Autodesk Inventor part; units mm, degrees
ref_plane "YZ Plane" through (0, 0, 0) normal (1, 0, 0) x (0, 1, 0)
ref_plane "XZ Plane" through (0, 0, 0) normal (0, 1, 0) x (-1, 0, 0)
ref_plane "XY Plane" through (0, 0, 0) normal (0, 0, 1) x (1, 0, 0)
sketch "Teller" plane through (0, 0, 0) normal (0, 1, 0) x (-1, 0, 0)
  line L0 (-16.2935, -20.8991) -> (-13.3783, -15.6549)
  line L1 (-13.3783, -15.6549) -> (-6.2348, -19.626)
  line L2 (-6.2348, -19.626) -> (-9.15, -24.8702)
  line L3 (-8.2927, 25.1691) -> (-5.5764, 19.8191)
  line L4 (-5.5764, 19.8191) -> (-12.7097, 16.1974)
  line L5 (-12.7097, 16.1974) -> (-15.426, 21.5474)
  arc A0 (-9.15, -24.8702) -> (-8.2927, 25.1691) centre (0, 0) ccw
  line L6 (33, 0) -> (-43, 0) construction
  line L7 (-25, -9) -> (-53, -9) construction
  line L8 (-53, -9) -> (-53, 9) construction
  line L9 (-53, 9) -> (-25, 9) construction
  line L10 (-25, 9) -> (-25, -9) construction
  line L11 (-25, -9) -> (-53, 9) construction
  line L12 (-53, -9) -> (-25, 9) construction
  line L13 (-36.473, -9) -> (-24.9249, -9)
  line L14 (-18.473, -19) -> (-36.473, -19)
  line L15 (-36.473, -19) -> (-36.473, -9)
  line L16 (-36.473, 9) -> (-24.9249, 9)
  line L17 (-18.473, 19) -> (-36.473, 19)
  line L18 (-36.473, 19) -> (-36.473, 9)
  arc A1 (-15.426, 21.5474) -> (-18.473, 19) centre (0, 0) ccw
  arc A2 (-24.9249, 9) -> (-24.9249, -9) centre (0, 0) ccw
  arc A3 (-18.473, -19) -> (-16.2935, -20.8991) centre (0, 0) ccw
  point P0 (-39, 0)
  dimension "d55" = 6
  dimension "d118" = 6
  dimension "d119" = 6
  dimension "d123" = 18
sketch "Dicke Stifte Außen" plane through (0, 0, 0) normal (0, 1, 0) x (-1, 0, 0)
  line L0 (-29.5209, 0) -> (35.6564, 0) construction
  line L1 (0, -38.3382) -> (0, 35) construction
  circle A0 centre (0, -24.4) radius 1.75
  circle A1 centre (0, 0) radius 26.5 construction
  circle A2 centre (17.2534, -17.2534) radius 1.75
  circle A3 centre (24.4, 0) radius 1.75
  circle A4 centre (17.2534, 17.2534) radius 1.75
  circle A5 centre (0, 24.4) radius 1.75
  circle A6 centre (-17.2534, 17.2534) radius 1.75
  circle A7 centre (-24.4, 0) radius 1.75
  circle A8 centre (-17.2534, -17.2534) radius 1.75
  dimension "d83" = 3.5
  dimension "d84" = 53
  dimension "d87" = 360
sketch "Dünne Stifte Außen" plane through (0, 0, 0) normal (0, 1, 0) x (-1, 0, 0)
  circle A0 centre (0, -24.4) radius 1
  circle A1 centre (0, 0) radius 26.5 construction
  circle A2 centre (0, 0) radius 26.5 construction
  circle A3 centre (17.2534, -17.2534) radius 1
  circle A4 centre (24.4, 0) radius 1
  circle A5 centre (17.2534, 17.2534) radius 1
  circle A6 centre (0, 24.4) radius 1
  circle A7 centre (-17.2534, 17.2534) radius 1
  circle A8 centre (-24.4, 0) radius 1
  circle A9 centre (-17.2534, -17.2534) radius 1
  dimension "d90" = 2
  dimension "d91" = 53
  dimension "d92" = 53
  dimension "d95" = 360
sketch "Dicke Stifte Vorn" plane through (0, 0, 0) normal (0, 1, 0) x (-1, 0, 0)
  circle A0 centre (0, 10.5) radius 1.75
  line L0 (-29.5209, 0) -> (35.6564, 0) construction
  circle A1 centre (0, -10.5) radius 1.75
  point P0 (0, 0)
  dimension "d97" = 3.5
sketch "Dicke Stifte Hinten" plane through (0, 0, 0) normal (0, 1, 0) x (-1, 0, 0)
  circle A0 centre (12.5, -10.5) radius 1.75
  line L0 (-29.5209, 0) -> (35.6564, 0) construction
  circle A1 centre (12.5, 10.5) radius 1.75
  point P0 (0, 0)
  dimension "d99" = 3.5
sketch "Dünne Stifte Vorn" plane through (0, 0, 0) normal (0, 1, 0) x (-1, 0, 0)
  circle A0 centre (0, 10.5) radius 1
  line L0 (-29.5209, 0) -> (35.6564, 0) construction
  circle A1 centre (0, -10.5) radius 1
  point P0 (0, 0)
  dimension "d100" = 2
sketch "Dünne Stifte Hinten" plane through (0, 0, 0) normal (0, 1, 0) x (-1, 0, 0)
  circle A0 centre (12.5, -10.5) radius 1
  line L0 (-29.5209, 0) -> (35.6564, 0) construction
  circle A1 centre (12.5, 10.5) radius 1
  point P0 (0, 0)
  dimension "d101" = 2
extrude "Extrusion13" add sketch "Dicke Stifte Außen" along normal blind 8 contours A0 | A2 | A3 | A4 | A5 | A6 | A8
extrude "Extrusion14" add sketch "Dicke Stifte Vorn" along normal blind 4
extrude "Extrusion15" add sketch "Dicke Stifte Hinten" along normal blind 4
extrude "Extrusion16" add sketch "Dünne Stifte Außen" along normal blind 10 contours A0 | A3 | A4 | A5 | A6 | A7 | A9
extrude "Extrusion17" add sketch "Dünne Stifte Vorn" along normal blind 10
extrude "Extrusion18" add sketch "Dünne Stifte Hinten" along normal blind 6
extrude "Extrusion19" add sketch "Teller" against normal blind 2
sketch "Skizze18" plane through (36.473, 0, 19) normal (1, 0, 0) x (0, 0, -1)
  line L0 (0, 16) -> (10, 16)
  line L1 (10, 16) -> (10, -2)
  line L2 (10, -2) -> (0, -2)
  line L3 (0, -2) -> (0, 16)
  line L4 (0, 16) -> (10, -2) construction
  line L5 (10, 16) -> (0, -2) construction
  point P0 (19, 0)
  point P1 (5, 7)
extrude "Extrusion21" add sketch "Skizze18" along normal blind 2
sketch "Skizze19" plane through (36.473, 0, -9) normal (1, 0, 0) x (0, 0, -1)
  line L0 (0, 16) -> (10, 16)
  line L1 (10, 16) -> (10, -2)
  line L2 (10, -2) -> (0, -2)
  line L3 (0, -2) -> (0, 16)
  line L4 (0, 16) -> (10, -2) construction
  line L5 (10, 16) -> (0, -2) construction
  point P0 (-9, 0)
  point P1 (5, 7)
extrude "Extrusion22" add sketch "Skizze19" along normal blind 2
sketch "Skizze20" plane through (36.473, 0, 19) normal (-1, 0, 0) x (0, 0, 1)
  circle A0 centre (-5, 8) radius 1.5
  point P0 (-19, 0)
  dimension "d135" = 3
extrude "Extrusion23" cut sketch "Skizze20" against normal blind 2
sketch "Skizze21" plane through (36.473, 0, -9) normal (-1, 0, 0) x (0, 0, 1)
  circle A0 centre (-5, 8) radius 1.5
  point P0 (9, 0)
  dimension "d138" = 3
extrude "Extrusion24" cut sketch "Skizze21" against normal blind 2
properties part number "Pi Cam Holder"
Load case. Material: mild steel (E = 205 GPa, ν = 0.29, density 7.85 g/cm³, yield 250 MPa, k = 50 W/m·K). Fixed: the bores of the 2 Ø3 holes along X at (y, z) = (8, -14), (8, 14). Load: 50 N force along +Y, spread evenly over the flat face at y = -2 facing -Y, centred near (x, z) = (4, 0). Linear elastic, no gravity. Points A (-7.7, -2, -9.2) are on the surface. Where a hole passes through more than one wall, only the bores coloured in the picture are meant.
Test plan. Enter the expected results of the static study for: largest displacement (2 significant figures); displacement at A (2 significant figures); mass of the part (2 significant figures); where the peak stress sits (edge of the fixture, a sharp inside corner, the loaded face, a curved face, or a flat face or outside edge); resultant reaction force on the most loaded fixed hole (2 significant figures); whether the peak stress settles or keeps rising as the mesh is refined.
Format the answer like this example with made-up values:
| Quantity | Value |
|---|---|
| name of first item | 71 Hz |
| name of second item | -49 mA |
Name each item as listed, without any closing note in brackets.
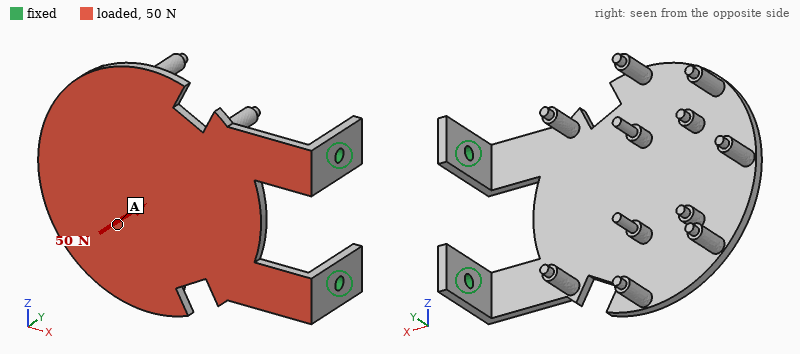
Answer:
| Quantity | Value |
|---|---|
| largest displacement | 0.82 mm |
| displacement at A | 0.54 mm |
| mass of the part | 49 g |
| where the peak stress sits | edge of the fixture |
| resultant reaction force on the most loaded fixed hole | 25 N |
| whether the peak stress settles or keeps rising as the mesh is refined | keeps rising |
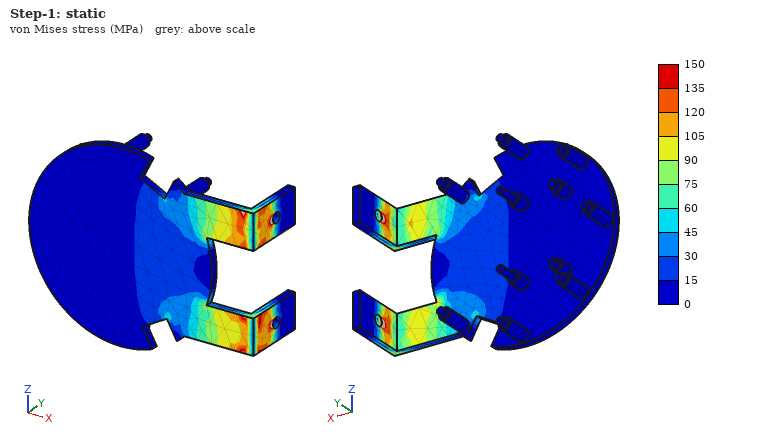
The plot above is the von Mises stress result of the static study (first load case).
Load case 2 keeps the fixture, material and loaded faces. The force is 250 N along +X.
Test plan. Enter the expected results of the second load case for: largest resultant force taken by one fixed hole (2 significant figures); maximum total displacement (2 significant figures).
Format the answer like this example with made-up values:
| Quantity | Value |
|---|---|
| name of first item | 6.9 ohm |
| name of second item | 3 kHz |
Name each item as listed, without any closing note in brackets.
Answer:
| Quantity | Value |
|---|---|
| largest resultant force taken by one fixed hole | 130 N |
| maximum total displacement | 0.35 mm |
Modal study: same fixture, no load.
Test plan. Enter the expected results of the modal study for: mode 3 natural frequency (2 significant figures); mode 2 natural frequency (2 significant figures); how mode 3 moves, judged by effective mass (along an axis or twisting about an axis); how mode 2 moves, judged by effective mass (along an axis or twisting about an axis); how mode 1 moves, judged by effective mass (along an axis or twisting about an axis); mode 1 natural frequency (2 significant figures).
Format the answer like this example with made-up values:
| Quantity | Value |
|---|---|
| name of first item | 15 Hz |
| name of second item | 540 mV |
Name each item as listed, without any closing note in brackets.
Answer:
| Quantity | Value |
|---|---|
| mode 3 natural frequency | 1300 Hz |
| mode 2 natural frequency | 850 Hz |
| how mode 3 moves, judged by effective mass | along Z |
| how mode 2 moves, judged by effective mass | along Z |
| how mode 1 moves, judged by effective mass | along Y |
| mode 1 natural frequency | 230 Hz |
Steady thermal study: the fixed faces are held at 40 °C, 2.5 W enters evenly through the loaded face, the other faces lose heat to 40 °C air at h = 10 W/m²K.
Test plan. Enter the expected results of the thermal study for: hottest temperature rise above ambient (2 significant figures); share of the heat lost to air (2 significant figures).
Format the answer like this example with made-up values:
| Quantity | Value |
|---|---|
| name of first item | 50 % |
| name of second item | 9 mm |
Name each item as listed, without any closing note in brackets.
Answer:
| Quantity | Value |
|---|---|
| hottest temperature rise above ambient | 26 K |
| share of the heat lost to air | 35 % |
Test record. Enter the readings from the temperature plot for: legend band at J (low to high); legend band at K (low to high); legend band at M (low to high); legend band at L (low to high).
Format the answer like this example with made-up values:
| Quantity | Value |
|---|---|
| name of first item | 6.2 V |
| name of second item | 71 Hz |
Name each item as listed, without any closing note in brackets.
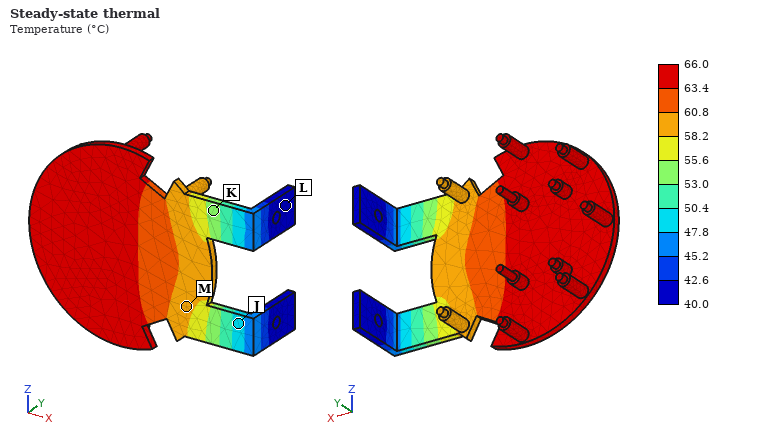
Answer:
| Quantity | Value |
|---|---|
| legend band at J | 47.8 to 50.4 °C |
| legend band at K | 53.0 to 55.6 °C |
| legend band at M | 58.2 to 60.8 °C |
| legend band at L | 40.0 to 42.6 °C |
